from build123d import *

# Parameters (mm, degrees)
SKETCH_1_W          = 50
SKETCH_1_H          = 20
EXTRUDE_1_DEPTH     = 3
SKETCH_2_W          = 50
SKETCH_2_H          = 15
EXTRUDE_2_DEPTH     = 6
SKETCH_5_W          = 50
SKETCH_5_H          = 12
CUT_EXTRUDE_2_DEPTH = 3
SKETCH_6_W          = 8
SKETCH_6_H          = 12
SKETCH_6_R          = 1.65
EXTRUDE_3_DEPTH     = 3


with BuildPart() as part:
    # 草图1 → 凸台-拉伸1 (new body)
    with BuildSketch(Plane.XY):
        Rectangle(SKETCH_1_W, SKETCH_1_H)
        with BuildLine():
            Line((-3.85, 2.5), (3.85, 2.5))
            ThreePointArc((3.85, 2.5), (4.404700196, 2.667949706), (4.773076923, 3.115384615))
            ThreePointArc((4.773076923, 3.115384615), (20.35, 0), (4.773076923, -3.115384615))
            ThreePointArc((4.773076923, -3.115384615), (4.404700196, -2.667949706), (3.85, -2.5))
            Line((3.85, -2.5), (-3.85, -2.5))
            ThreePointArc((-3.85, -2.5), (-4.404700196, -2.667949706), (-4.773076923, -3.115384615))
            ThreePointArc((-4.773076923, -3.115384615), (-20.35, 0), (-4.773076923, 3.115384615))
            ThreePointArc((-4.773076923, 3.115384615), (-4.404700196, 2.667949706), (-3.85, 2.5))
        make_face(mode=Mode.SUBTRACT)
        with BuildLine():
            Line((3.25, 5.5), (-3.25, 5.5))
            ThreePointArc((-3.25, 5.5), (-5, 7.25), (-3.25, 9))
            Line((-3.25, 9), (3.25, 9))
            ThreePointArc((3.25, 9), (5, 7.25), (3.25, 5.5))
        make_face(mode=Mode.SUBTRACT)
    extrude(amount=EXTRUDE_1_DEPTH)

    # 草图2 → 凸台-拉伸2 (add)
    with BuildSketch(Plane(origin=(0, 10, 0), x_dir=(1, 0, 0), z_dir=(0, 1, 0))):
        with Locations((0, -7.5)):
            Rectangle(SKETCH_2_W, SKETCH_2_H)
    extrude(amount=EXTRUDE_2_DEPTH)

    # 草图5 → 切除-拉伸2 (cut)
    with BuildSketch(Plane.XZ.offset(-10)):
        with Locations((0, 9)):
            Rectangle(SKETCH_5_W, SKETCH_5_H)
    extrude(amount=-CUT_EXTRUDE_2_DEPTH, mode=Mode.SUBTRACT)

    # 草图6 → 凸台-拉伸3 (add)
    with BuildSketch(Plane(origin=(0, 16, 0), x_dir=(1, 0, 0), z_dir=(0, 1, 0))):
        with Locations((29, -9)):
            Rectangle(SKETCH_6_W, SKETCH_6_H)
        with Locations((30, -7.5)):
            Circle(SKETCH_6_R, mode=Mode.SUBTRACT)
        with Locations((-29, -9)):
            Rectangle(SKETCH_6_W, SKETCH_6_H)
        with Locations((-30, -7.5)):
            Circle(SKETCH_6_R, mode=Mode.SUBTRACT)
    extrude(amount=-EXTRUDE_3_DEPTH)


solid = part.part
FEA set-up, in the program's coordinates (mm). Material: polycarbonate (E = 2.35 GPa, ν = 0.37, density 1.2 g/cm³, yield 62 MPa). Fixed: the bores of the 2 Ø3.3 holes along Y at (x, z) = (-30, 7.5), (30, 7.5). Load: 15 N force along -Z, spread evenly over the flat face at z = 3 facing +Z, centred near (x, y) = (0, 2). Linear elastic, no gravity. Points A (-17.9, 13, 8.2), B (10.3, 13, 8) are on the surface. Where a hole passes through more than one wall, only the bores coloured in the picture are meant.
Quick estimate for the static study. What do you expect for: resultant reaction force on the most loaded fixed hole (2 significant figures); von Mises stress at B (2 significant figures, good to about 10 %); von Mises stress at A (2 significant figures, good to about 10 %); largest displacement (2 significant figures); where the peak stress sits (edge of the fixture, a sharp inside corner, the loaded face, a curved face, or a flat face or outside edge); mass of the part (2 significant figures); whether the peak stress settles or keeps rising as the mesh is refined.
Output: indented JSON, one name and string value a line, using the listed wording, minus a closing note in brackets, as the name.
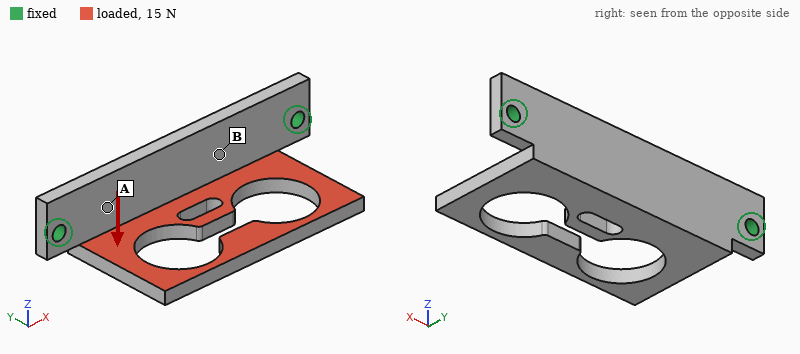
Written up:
{
  "resultant reaction force on the most loaded fixed hole": "7.6 N",
  "von Mises stress at B": "1.2 MPa",
  "von Mises stress at A": "2.5 MPa",
  "largest displacement": "0.72 mm",
  "where the peak stress sits": "edge of the fixture",
  "mass of the part": "5.7 g",
  "whether the peak stress settles or keeps rising as the mesh is refined": "keeps rising"
}
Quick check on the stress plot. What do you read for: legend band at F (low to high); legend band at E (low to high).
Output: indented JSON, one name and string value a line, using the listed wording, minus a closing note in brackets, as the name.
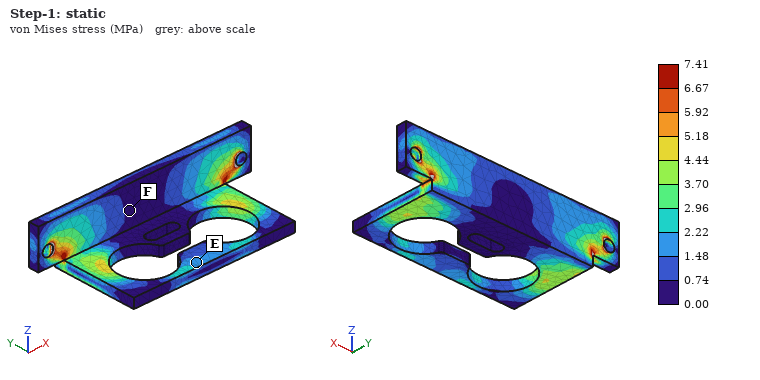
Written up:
{
  "legend band at F": "0.00 to 0.74 MPa",
  "legend band at E": "1.48 to 2.22 MPa"
}
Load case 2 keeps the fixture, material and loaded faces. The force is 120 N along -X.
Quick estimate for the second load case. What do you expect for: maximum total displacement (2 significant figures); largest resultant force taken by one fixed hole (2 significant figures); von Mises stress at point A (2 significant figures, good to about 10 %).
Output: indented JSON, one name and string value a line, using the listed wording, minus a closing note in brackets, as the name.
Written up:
{
  "maximum total displacement": "0.71 mm",
  "largest resultant force taken by one fixed hole": "67 N",
  "von Mises stress at point A": "3.1 MPa"
}
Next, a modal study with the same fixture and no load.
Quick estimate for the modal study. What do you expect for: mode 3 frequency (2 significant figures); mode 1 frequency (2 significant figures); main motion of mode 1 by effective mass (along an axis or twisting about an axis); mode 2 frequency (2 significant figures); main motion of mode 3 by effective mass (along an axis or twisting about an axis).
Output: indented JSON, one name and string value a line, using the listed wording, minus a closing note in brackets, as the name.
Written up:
{
  "mode 3 frequency": "1600 Hz",
  "mode 1 frequency": "560 Hz",
  "main motion of mode 1 by effective mass": "along Z",
  "mode 2 frequency": "1100 Hz",
  "main motion of mode 3 by effective mass": "along Y"
}
